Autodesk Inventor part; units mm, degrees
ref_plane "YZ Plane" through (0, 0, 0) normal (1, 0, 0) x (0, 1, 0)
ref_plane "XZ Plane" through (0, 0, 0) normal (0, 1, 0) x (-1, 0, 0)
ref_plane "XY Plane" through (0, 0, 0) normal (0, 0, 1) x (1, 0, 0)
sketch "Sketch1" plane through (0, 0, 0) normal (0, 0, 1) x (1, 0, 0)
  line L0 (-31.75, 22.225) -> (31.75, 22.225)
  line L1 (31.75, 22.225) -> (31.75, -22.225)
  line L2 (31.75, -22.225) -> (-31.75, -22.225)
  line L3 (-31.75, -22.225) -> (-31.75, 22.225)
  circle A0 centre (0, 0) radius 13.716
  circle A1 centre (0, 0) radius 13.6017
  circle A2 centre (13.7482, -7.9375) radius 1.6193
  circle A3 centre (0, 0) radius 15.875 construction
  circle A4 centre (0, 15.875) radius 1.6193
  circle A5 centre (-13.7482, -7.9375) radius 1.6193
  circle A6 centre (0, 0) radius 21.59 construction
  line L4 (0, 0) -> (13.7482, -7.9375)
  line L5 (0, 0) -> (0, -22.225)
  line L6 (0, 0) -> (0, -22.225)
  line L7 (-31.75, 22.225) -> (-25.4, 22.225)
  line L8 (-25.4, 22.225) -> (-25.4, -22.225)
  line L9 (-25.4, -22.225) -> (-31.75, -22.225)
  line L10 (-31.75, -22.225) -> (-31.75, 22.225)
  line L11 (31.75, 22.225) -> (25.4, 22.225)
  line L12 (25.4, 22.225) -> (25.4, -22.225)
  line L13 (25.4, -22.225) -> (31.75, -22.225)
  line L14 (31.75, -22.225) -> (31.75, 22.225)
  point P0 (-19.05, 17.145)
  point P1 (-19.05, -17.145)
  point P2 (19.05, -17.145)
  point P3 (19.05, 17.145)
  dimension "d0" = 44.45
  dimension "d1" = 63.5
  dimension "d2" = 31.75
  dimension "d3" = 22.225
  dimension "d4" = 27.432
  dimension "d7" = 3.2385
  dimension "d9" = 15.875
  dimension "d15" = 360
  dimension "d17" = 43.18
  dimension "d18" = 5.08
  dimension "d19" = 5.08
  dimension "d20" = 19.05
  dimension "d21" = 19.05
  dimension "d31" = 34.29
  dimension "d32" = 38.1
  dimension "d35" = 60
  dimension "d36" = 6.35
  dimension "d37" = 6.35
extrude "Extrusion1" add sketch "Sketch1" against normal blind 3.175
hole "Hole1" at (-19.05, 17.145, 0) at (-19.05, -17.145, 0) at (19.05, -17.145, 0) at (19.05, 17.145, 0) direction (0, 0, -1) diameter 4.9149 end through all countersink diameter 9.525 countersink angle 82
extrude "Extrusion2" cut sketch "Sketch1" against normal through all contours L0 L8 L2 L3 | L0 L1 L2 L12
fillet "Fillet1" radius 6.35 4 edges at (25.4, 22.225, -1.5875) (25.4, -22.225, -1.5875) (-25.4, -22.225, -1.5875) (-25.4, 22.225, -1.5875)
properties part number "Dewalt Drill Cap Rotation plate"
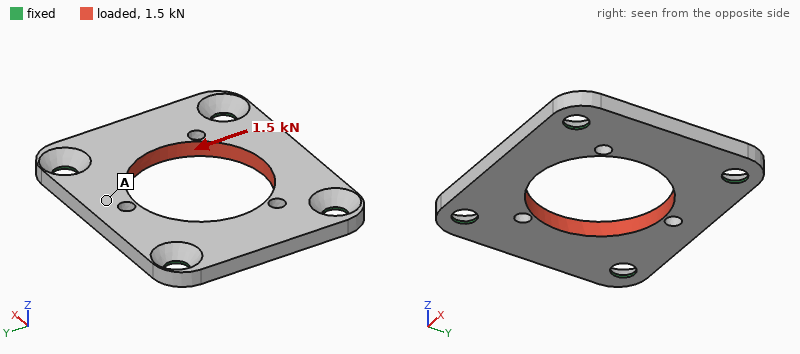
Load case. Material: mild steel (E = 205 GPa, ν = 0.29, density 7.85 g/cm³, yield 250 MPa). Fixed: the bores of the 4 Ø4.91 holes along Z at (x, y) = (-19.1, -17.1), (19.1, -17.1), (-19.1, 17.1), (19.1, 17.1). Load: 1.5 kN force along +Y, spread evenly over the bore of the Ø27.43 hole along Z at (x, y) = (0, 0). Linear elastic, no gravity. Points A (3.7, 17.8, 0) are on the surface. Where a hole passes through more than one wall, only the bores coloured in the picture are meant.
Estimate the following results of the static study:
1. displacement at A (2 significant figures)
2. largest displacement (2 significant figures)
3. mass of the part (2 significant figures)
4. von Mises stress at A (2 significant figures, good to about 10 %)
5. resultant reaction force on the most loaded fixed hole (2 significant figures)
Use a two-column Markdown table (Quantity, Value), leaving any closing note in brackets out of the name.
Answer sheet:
| Quantity | Value |
|---|---|
| displacement at A | 2.5 µm |
| largest displacement | 3.2 µm |
| mass of the part | 36 g |
| von Mises stress at A | 9.8 MPa |
| resultant reaction force on the most loaded fixed hole | 380 N |
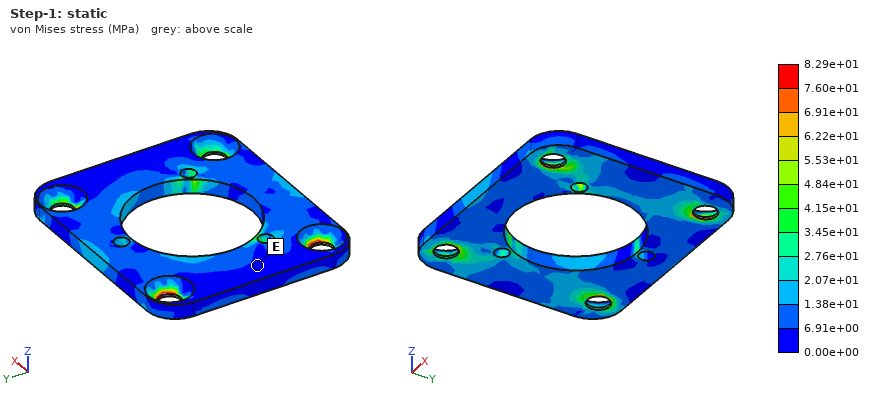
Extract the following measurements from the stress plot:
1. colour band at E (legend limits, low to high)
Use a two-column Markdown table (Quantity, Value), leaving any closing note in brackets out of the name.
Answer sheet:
| Quantity | Value |
|---|---|
| colour band at E | 0.00e+00 to 6.91e+00 MPa |
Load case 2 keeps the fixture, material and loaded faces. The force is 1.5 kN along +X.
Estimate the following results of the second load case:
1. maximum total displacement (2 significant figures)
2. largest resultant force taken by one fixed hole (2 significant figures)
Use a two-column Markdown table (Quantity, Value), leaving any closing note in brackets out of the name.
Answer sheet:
| Quantity | Value |
|---|---|
| maximum total displacement | 2.6 µm |
| largest resultant force taken by one fixed hole | 380 N |
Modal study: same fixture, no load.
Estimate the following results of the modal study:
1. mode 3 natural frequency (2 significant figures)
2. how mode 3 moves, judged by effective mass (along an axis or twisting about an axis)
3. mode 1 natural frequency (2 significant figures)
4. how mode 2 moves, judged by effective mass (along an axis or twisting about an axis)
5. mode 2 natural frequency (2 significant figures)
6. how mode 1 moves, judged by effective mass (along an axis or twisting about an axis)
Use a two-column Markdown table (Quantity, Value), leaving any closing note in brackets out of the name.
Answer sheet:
| Quantity | Value |
|---|---|
| mode 3 natural frequency | 11 kHz |
| how mode 3 moves, judged by effective mass | along Z |
| mode 1 natural frequency | 9600 Hz |
| how mode 2 moves, judged by effective mass | twisting about X |
| mode 2 natural frequency | 11 kHz |
| how mode 1 moves, judged by effective mass | along Z |
